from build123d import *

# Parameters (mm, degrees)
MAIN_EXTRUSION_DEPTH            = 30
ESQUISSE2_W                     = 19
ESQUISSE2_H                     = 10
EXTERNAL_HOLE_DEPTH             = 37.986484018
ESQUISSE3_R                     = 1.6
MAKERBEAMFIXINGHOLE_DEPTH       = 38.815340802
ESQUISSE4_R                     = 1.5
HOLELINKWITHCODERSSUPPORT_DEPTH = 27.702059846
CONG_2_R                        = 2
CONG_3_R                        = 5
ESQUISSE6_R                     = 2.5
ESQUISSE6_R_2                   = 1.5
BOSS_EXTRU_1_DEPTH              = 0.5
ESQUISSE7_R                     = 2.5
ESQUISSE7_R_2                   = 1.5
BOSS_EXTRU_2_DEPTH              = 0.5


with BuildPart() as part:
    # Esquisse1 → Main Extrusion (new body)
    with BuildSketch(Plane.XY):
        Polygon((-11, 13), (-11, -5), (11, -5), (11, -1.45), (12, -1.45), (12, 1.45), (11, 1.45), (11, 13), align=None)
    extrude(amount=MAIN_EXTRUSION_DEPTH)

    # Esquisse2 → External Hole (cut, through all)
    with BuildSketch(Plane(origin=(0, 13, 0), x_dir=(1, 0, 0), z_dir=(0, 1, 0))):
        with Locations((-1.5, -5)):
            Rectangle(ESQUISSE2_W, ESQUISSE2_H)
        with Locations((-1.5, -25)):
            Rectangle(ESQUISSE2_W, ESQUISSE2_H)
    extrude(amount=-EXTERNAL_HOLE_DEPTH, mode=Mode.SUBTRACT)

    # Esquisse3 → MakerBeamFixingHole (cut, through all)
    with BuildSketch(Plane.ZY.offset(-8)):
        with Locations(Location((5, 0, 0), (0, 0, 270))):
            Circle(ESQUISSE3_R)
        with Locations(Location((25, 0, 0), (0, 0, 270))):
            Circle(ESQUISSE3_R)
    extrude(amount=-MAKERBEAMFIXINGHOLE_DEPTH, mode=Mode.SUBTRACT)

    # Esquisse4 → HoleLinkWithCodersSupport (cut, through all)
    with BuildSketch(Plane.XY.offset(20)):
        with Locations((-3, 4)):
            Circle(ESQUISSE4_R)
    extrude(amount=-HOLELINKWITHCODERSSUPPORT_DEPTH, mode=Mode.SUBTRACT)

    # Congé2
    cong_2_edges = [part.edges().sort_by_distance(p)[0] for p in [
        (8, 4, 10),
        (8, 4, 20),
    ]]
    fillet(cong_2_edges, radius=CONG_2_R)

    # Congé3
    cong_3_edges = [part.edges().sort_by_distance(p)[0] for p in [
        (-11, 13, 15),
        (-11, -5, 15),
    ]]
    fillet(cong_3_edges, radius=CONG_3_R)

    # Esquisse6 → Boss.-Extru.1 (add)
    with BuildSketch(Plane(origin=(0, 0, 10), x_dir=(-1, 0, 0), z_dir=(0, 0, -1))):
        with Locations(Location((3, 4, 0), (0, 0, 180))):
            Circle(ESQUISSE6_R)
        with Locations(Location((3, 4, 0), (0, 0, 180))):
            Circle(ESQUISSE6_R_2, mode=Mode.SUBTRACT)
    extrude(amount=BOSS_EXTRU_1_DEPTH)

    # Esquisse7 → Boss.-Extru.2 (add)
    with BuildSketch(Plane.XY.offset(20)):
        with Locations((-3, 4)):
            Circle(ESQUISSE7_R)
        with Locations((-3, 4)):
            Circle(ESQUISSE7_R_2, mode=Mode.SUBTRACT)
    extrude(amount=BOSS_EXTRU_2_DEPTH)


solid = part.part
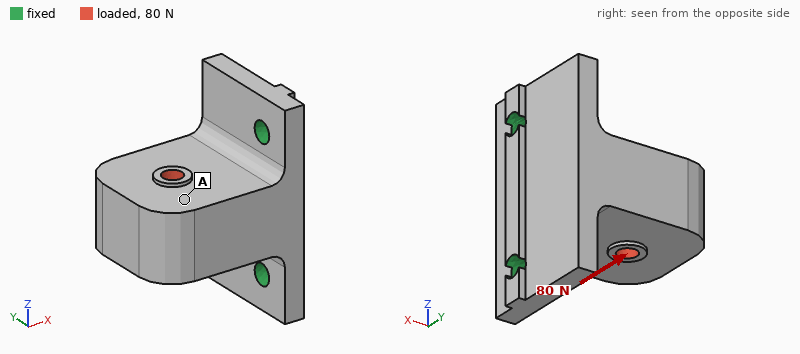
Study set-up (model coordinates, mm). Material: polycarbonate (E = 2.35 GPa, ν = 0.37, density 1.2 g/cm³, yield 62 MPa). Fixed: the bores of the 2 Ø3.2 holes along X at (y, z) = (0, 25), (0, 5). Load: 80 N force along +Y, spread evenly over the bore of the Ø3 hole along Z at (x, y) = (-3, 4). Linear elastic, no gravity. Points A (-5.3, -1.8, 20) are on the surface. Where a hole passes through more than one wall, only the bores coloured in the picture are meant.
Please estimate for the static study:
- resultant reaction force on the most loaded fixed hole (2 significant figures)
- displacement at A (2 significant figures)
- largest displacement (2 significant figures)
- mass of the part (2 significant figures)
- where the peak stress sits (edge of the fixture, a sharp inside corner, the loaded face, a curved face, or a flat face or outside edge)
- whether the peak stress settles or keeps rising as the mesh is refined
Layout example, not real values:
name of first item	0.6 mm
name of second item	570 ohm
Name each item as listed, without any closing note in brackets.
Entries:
resultant reaction force on the most loaded fixed hole	44 N
displacement at A	0.27 mm
largest displacement	0.39 mm
mass of the part	5.9 g
where the peak stress sits	edge of the fixture
whether the peak stress settles or keeps rising as the mesh is refined	keeps rising
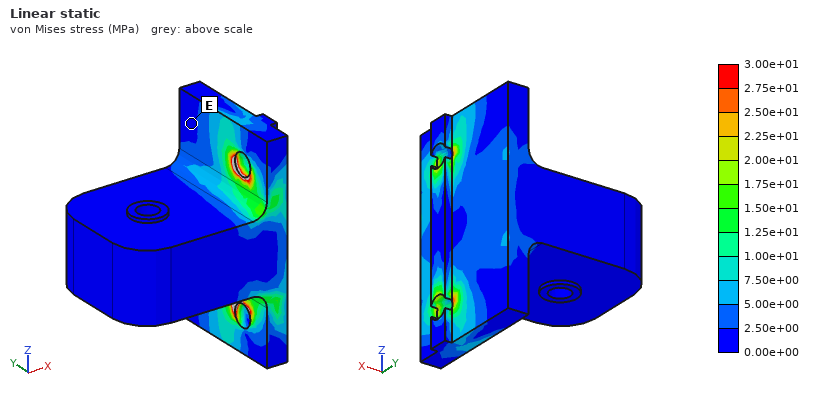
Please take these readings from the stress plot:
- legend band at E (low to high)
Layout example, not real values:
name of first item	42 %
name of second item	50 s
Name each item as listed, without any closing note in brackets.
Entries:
legend band at E	0.00e+00 to 2.50e+00 MPa
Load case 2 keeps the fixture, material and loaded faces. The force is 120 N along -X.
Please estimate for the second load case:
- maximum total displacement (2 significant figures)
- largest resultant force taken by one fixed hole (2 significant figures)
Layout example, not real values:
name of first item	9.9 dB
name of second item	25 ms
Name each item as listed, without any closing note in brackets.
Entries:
maximum total displacement	0.17 mm
largest resultant force taken by one fixed hole	64 N
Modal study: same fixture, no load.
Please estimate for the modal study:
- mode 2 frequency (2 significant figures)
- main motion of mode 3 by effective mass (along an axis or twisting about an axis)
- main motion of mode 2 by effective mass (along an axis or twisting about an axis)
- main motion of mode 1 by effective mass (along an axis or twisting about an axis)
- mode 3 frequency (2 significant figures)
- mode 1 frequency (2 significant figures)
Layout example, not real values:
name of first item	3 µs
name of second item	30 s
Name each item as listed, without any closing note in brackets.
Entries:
mode 2 frequency	3100 Hz
main motion of mode 3 by effective mass	along X
main motion of mode 2 by effective mass	along Z
main motion of mode 1 by effective mass	along Y
mode 3 frequency	5400 Hz
mode 1 frequency	1400 Hz
